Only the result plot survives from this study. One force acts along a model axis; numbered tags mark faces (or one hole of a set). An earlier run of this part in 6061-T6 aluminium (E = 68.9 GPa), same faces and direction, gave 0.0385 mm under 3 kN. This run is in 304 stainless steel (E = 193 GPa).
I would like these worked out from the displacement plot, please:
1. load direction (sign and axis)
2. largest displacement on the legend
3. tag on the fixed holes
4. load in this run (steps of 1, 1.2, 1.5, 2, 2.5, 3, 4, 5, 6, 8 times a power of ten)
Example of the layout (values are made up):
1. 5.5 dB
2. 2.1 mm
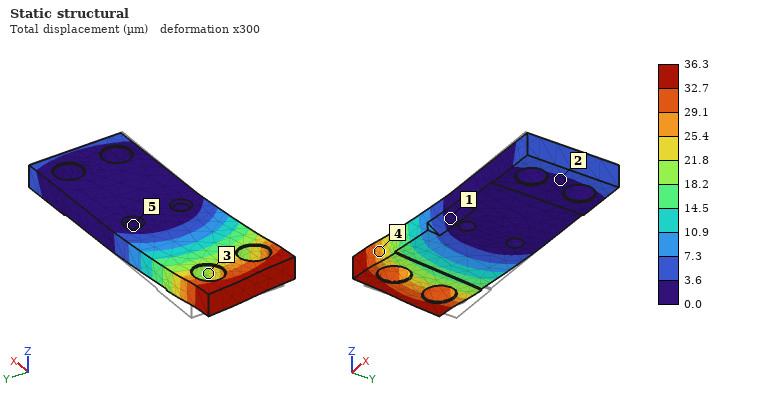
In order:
1. -Y
2. 36.3 µm
3. 5
4. 8 kN
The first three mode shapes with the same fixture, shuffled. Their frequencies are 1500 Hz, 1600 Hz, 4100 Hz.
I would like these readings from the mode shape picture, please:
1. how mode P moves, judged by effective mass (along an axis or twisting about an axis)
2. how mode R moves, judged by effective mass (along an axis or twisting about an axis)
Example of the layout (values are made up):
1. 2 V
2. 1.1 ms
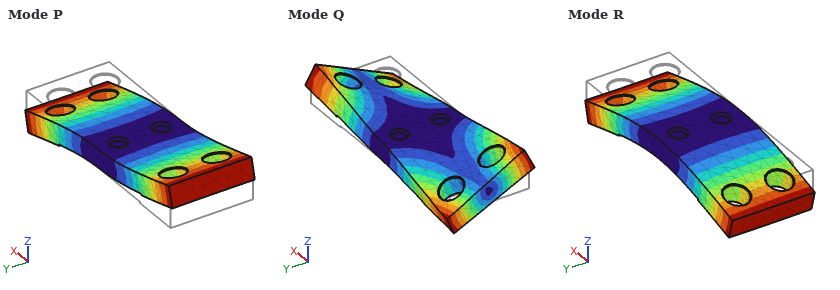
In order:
1. twisting about Y
2. along Z
